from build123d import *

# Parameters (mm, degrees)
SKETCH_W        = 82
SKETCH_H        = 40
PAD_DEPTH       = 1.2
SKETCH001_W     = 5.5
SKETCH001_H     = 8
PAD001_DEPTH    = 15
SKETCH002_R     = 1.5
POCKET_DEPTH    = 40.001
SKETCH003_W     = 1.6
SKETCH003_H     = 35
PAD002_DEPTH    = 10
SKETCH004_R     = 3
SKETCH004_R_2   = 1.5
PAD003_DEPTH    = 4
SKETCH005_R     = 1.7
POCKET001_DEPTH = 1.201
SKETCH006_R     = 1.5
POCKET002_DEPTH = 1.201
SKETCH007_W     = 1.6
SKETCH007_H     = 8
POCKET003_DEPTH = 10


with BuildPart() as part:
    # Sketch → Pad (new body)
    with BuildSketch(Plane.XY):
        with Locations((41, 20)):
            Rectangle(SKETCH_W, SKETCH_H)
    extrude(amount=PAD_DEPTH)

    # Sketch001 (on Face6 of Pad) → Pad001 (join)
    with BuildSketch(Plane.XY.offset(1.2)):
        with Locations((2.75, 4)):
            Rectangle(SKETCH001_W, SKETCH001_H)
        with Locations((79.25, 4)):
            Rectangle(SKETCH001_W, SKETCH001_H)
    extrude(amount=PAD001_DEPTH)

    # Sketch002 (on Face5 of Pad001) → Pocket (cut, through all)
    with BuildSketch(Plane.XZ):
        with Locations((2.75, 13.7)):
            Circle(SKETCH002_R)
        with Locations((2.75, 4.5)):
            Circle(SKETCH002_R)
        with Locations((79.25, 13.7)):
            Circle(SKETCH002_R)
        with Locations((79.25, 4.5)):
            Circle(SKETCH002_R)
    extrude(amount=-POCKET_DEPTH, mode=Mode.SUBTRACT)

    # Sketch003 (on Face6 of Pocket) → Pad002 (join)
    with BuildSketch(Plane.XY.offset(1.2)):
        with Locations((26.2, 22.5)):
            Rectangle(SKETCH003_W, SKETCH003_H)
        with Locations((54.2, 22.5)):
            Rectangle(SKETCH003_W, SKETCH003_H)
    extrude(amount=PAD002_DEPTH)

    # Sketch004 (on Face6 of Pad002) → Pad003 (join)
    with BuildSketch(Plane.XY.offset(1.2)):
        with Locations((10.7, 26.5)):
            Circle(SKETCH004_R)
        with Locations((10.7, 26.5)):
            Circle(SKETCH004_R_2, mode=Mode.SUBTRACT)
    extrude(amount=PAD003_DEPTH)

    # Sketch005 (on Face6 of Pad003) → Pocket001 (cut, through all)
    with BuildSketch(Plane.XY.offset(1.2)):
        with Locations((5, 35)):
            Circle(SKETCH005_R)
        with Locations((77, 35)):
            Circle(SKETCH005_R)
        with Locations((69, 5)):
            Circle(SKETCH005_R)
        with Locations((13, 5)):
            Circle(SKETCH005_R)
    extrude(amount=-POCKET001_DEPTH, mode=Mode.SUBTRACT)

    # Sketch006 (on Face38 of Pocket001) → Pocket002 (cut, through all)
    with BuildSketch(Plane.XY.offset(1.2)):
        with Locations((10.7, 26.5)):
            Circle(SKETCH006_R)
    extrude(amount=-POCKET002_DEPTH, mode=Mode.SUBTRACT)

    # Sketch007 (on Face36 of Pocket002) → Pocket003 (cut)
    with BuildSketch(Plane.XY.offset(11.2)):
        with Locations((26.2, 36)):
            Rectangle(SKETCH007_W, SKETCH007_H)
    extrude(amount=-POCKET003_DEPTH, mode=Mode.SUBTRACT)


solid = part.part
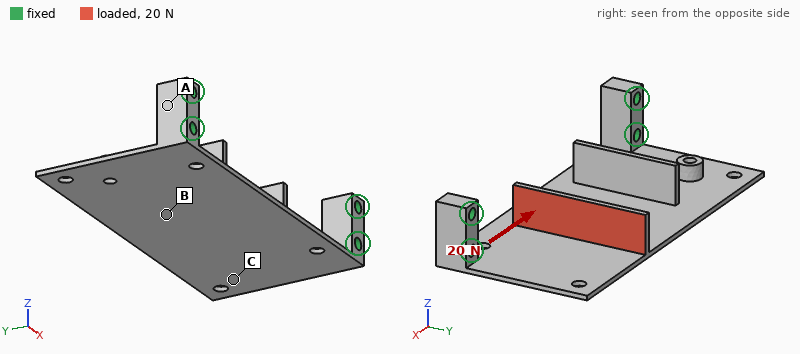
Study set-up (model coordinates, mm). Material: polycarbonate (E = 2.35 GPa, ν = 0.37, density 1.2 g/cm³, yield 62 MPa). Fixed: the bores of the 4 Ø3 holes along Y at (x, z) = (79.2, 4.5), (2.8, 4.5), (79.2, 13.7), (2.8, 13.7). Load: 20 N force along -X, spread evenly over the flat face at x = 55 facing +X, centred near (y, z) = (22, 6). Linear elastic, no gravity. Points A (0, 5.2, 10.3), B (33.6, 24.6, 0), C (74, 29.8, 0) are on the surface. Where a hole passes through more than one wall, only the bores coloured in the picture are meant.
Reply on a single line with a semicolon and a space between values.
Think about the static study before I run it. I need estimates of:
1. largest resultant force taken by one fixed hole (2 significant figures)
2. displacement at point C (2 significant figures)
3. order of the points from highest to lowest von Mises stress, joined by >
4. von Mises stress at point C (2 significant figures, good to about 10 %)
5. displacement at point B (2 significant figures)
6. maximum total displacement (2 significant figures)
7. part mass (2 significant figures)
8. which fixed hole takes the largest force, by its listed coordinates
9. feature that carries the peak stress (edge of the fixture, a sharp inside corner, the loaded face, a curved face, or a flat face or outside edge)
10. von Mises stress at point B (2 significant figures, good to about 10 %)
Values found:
13 N; 0.32 mm; B > C > A; 2.0 MPa; 0.83 mm; 1.0 mm; 7.3 g; (79.2, 4.5); a flat face or outside edge; 2.7 MPa
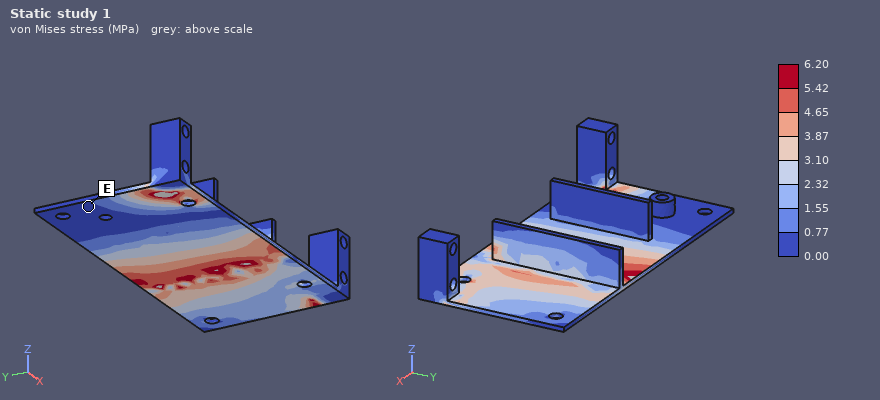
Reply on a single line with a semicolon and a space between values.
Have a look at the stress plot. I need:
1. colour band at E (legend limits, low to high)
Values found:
0.00 to 0.77 MPa
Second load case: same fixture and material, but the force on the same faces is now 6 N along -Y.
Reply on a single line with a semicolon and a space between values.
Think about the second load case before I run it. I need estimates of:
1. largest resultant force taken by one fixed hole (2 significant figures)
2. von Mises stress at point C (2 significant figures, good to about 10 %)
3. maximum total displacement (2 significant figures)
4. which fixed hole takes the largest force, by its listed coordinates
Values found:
4.4 N; 0.35 MPa; 1.0 mm; (79.2, 4.5)
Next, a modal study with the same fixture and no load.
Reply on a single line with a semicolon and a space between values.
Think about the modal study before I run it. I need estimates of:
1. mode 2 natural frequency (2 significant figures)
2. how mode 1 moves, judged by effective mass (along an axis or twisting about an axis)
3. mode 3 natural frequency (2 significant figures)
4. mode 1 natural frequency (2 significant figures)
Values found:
310 Hz; along Z; 320 Hz; 130 Hz
